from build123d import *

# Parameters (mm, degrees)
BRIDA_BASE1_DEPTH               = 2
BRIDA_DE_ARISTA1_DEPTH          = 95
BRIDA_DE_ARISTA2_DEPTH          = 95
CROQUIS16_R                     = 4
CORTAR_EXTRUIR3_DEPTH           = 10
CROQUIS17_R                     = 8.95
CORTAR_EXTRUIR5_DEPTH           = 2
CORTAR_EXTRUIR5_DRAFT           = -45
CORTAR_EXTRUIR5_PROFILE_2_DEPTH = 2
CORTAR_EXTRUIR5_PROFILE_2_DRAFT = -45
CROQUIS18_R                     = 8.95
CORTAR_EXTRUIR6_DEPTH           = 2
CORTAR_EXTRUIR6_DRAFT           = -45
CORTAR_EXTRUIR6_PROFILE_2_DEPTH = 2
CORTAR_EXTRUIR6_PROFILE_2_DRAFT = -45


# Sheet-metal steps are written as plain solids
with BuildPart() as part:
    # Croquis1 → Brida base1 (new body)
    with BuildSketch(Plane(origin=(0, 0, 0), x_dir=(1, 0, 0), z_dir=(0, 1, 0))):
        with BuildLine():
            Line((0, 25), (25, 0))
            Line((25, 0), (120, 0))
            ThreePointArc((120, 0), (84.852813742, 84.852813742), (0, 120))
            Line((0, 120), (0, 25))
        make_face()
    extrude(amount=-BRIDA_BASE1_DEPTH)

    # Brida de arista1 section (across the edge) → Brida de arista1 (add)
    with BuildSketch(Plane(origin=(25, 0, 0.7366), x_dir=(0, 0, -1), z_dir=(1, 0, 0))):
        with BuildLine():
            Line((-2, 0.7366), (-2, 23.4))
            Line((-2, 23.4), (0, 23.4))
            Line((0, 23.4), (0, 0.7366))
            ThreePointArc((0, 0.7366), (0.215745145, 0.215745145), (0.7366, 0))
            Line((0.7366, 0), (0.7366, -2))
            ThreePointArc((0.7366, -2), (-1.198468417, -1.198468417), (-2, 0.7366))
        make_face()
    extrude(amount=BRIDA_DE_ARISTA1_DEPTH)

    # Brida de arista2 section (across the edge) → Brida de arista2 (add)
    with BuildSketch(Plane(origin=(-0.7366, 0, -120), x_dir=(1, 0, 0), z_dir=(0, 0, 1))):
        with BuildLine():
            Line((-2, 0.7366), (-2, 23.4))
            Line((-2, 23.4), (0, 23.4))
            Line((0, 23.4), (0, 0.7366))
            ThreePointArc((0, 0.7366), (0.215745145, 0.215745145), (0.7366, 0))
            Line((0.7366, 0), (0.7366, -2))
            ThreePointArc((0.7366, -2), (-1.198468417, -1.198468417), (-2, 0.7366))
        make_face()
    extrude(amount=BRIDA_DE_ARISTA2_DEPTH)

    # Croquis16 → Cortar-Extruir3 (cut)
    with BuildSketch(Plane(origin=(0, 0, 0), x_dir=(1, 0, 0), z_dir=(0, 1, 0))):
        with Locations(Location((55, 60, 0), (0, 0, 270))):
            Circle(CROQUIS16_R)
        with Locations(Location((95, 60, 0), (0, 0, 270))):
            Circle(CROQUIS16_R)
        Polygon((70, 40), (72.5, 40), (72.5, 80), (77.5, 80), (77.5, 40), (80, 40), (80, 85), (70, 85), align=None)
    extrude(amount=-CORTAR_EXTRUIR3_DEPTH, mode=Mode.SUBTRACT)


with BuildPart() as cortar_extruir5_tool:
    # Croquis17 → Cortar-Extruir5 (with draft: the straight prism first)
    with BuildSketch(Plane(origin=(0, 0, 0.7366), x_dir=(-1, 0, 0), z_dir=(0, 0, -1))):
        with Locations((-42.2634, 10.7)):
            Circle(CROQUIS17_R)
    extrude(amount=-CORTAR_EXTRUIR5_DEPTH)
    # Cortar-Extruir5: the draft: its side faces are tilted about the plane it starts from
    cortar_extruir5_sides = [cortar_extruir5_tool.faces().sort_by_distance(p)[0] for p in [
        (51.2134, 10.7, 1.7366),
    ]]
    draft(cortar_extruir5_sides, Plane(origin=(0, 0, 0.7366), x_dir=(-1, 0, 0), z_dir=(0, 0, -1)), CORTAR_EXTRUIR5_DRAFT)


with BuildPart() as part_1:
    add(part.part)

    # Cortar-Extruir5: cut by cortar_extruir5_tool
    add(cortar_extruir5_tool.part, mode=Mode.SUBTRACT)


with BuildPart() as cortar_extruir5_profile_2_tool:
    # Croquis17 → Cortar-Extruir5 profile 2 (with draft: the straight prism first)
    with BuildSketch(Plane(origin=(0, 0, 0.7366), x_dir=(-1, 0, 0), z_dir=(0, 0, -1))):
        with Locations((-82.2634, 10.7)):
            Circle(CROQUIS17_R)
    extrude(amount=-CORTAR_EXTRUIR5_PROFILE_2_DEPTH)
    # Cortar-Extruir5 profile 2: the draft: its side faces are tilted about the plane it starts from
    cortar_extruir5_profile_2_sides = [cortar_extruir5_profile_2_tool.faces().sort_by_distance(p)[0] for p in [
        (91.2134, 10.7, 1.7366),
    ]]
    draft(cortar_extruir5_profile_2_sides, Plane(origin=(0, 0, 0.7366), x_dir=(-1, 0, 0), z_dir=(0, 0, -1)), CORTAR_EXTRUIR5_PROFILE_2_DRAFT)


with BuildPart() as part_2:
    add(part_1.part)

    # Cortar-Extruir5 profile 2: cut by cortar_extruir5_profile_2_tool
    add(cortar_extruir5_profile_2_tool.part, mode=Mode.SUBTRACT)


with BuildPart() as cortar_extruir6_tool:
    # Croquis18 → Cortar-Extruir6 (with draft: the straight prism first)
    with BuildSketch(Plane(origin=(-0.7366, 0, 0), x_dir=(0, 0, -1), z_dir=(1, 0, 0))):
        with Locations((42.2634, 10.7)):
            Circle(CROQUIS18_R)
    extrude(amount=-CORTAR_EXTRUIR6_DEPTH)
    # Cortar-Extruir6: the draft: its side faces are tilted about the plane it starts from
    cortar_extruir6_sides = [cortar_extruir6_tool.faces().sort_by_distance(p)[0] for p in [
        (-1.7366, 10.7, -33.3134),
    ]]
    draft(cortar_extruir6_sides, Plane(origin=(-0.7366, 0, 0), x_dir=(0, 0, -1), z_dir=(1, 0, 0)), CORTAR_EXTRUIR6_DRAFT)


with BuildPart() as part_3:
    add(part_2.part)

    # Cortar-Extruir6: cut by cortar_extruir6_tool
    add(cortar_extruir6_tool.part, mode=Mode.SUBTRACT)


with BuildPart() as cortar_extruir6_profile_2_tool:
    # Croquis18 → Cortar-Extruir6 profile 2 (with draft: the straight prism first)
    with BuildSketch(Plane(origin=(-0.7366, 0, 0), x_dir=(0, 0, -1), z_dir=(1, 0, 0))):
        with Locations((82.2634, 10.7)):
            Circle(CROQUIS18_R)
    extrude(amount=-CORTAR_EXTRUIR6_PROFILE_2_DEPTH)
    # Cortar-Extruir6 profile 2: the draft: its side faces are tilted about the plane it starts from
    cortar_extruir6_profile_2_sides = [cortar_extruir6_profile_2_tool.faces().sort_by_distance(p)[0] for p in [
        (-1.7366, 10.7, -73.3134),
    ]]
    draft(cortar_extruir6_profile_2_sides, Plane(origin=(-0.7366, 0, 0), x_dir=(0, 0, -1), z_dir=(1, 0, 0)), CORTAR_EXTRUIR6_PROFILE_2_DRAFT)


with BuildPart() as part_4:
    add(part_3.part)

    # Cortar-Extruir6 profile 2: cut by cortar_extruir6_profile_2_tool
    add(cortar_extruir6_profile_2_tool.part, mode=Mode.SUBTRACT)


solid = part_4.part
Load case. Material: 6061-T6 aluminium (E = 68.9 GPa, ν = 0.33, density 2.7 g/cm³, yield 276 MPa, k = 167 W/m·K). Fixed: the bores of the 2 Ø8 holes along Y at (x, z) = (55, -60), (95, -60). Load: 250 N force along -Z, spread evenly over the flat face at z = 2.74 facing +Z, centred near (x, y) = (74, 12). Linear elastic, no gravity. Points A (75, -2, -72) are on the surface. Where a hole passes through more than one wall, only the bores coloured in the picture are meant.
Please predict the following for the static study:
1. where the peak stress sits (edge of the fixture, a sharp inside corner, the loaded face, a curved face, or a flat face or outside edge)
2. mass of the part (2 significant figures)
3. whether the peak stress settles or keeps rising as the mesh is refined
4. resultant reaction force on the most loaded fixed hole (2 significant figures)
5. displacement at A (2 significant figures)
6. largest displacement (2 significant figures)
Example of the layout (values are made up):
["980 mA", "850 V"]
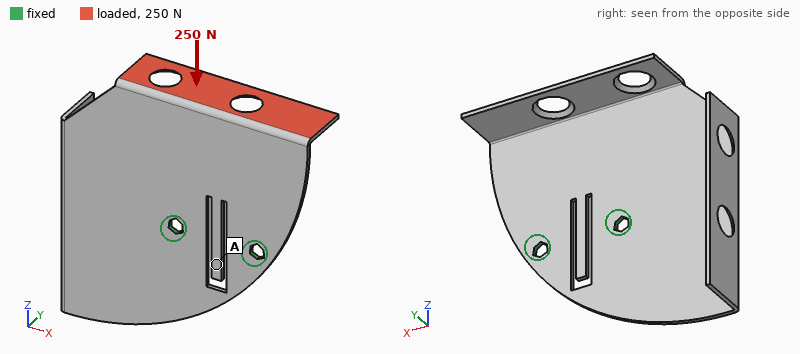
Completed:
["edge of the fixture", "79 g", "keeps rising", "130 N", "0.45 mm", "1.9 mm"]
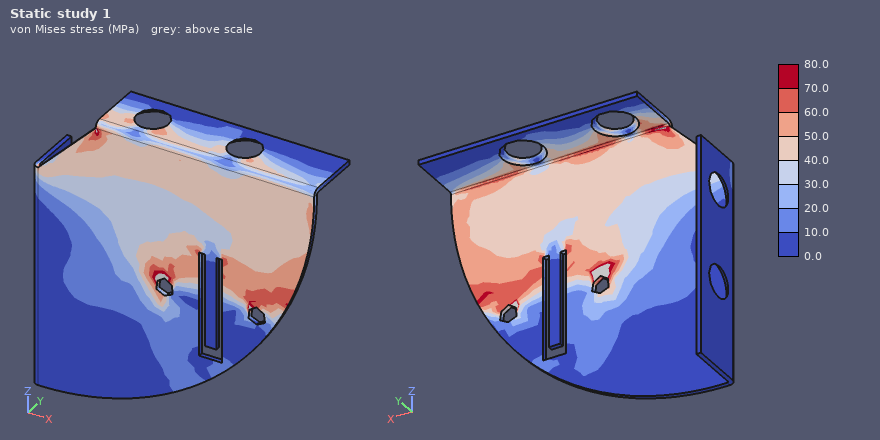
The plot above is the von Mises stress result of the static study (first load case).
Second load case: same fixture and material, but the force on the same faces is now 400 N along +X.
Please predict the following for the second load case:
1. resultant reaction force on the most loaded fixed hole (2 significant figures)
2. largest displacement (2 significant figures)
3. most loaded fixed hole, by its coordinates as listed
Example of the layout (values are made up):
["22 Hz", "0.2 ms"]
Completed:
["560 N", "1.8 mm", "(55, -60)"]
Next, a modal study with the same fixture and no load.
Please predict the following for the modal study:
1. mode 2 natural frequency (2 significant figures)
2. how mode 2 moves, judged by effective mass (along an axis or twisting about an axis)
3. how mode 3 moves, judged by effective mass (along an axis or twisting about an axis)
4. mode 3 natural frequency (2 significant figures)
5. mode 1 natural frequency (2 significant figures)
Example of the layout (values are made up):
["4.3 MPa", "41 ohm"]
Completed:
["300 Hz", "along Y", "twisting about Z", "390 Hz", "250 Hz"]
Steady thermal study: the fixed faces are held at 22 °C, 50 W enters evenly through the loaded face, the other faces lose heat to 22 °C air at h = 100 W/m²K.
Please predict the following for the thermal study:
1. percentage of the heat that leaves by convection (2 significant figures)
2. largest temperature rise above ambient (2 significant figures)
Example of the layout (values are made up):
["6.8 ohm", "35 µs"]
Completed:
["78 %", "65 K"]
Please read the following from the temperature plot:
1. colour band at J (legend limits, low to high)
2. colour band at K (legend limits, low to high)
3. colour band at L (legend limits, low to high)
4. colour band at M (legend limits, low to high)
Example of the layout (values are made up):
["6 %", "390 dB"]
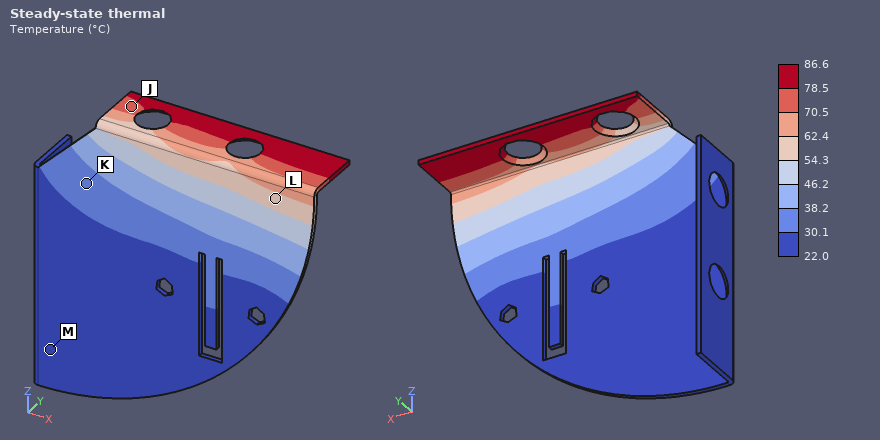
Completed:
["70.5 to 78.5 °C", "30.1 to 38.2 °C", "54.3 to 62.4 °C", "22.0 to 30.1 °C"]
